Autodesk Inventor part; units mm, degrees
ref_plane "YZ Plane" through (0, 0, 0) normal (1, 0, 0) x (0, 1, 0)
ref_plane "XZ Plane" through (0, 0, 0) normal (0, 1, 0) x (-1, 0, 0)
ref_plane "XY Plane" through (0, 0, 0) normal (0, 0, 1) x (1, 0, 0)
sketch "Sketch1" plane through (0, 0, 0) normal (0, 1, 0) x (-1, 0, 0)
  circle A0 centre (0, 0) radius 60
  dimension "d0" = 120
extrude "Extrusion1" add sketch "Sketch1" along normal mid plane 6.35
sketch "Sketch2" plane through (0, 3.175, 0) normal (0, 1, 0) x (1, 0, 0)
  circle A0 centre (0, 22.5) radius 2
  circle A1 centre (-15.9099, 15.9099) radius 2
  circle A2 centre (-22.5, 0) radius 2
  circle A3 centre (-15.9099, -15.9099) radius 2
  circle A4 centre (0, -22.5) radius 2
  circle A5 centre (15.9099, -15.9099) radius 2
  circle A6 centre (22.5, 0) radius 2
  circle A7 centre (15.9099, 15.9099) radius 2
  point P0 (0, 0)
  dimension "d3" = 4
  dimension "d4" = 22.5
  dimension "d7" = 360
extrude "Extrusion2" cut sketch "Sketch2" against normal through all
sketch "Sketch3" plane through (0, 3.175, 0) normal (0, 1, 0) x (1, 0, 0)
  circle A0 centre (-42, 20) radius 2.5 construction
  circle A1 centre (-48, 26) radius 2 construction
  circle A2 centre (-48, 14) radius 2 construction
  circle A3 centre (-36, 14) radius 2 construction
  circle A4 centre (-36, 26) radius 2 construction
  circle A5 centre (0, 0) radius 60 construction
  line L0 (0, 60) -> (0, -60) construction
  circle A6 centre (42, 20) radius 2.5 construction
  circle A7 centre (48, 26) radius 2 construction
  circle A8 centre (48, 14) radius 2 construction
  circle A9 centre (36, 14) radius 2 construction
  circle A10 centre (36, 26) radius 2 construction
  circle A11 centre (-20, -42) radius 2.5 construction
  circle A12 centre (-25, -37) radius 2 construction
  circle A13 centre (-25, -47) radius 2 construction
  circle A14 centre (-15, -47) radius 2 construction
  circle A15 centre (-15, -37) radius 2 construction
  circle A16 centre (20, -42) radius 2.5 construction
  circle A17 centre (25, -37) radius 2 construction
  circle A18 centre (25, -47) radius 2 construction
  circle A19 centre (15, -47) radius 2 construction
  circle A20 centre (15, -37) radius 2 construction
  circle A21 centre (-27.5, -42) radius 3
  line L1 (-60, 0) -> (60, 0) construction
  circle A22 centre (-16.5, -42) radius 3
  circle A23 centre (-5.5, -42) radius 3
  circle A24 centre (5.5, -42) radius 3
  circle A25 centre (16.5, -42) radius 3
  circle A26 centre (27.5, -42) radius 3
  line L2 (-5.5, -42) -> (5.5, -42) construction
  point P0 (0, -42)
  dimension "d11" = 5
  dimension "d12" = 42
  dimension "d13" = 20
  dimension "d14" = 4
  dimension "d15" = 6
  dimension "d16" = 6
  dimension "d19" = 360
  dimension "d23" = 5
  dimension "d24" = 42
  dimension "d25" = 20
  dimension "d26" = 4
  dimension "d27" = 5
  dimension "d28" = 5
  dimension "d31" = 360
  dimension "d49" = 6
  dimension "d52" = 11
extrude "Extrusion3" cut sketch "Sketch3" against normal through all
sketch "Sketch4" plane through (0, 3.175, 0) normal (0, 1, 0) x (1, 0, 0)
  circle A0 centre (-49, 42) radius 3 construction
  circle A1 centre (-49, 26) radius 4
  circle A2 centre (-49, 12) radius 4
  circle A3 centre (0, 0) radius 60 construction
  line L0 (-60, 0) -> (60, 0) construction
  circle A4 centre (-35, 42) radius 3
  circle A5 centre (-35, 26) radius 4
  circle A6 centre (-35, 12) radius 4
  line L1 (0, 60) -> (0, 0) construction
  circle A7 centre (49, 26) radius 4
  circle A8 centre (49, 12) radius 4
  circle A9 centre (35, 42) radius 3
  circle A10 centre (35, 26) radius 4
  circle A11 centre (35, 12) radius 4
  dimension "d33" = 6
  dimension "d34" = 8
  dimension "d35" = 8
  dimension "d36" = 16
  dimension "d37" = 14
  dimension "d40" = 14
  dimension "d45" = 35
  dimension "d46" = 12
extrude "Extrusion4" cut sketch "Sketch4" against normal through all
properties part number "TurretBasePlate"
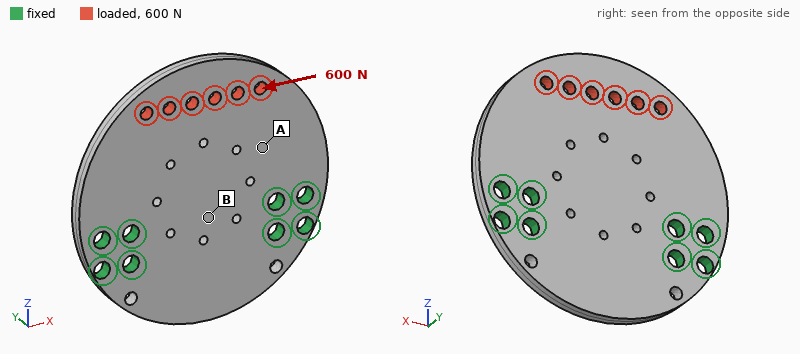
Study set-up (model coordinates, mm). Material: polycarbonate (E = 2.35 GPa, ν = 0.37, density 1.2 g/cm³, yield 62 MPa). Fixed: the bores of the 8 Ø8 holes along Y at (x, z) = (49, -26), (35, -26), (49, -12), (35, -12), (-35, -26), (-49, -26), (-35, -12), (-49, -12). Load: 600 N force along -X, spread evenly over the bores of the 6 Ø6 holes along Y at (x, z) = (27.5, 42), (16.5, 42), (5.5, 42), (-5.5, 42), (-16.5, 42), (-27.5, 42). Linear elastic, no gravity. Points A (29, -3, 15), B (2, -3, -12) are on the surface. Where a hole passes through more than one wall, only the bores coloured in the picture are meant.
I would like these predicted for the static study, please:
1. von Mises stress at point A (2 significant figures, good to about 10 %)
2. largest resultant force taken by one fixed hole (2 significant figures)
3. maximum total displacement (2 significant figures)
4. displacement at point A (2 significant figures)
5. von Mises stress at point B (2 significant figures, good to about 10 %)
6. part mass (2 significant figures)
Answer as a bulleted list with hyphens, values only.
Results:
- 1.8 MPa
- 250 N
- 89 µm
- 34 µm
- 0.67 MPa
- 81 g
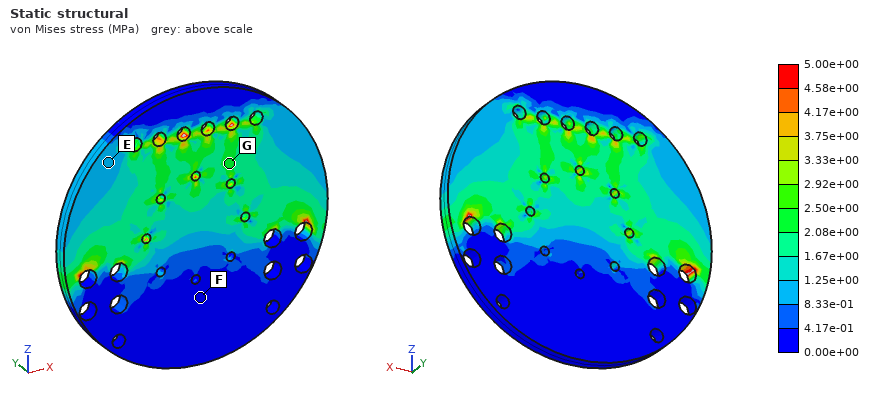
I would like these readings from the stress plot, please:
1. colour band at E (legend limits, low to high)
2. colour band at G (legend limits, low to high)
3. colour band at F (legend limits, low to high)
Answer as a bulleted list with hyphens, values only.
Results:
- 8.33e-01 to 1.25e+00 MPa
- 2.08e+00 to 2.50e+00 MPa
- 0.00e+00 to 4.17e-01 MPa
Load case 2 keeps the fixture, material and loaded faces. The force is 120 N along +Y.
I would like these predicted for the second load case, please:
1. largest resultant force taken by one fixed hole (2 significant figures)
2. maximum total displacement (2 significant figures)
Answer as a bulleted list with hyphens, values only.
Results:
- 120 N
- 1.8 mm
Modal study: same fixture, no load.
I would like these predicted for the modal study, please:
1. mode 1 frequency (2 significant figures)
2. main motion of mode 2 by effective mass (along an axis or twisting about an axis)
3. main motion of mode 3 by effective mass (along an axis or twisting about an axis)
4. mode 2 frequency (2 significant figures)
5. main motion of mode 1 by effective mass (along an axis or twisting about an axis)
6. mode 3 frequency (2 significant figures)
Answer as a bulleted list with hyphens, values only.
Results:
- 360 Hz
- twisting about Z
- along Y
- 810 Hz
- along Y
- 1200 Hz
